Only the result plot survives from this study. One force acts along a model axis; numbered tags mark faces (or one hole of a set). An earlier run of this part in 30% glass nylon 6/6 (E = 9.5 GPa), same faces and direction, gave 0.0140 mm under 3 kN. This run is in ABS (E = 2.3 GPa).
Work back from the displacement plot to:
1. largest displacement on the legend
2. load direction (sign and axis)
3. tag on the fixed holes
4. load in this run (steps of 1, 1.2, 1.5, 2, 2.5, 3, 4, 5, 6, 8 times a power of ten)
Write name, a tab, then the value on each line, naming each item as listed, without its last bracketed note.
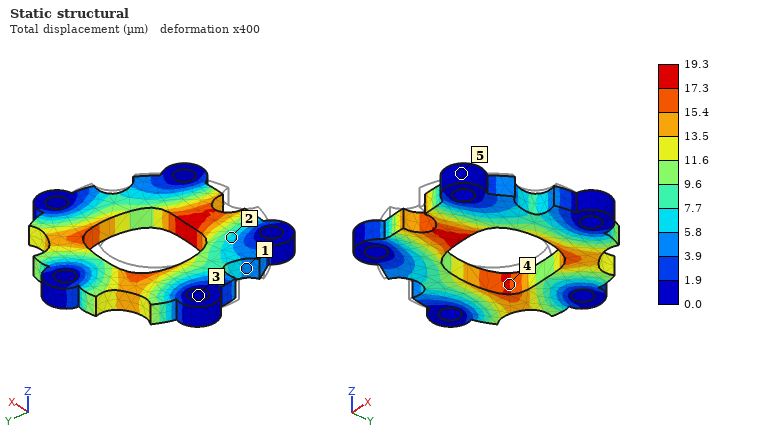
largest displacement on the legend	19.3 µm
load direction	+Y
tag on the fixed holes	3
load in this run	1 kN
